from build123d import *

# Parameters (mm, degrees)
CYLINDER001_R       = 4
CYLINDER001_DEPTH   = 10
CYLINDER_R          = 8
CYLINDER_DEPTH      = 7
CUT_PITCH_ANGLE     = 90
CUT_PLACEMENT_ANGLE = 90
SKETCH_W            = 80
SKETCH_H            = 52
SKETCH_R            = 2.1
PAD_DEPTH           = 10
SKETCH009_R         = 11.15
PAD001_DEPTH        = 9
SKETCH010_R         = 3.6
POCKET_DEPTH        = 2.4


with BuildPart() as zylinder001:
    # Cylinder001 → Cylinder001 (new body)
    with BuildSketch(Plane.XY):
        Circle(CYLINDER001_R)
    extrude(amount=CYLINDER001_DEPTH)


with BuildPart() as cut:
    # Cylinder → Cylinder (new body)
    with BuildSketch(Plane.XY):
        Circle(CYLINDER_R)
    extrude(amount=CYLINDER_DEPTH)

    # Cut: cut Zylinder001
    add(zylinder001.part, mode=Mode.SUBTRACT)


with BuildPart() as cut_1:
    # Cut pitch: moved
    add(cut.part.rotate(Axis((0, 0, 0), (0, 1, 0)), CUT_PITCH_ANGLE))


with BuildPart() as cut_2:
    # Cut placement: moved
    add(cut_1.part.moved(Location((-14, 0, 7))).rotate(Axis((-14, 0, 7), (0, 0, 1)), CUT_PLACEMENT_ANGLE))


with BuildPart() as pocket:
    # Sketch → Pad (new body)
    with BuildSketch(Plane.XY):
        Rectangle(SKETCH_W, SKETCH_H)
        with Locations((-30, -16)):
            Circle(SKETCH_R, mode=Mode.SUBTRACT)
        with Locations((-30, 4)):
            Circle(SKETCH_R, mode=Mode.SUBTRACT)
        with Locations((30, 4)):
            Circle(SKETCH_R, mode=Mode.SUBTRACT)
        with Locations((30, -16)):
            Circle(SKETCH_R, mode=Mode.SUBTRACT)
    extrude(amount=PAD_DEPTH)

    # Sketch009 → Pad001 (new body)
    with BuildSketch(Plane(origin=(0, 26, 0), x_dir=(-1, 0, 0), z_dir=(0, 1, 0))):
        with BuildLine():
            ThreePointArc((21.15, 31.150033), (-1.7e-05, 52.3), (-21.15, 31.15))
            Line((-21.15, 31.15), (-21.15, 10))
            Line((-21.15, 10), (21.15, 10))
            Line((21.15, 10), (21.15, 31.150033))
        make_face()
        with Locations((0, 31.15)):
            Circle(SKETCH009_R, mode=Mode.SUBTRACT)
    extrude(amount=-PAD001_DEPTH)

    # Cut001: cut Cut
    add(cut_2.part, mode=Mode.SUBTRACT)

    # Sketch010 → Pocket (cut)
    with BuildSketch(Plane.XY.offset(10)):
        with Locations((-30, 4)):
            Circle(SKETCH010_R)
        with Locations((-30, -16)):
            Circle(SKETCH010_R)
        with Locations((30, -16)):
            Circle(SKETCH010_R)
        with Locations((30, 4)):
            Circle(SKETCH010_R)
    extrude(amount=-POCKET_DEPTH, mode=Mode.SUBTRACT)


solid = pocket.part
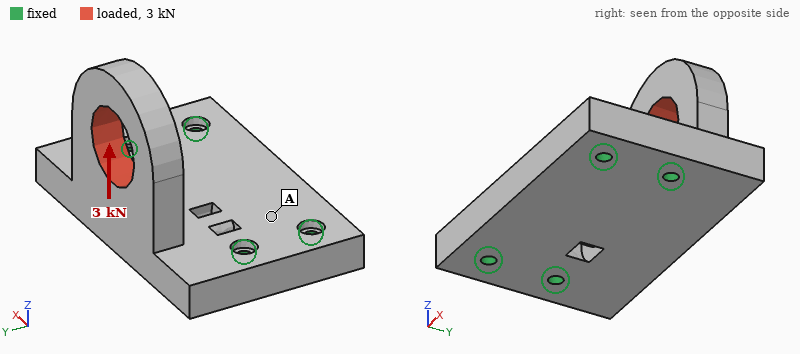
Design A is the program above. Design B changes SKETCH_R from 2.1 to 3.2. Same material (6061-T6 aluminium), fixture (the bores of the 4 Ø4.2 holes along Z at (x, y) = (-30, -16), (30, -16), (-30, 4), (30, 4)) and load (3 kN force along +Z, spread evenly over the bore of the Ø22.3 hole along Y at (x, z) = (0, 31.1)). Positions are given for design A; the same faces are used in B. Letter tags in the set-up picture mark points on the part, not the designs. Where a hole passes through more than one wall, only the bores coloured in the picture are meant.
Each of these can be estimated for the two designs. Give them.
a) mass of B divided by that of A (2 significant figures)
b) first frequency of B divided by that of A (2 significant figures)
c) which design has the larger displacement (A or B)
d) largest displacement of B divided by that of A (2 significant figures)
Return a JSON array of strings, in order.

["0.99", "1.0", "A", "0.85"]
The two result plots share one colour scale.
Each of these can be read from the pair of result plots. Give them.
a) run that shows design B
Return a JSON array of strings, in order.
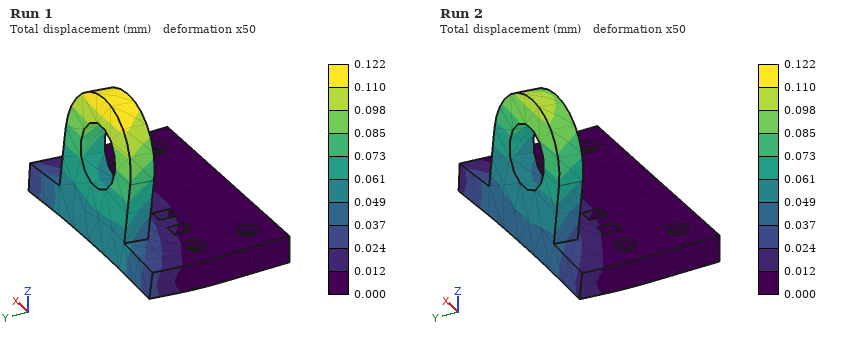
["Run 2"]
